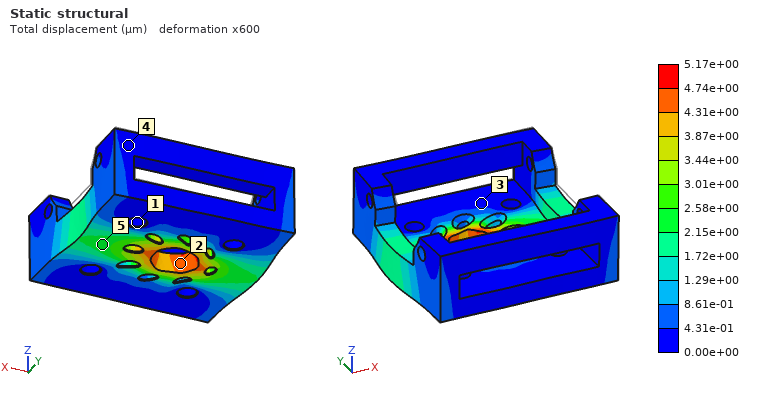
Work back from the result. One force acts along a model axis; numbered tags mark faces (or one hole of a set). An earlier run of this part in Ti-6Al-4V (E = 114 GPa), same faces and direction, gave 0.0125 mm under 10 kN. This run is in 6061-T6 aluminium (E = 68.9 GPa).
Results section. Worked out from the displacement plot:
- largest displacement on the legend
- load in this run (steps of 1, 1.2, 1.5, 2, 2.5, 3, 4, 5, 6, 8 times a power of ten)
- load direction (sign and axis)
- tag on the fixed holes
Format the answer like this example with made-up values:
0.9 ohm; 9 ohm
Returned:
5.17e+00 µm; 2.5 kN; -X; 1
